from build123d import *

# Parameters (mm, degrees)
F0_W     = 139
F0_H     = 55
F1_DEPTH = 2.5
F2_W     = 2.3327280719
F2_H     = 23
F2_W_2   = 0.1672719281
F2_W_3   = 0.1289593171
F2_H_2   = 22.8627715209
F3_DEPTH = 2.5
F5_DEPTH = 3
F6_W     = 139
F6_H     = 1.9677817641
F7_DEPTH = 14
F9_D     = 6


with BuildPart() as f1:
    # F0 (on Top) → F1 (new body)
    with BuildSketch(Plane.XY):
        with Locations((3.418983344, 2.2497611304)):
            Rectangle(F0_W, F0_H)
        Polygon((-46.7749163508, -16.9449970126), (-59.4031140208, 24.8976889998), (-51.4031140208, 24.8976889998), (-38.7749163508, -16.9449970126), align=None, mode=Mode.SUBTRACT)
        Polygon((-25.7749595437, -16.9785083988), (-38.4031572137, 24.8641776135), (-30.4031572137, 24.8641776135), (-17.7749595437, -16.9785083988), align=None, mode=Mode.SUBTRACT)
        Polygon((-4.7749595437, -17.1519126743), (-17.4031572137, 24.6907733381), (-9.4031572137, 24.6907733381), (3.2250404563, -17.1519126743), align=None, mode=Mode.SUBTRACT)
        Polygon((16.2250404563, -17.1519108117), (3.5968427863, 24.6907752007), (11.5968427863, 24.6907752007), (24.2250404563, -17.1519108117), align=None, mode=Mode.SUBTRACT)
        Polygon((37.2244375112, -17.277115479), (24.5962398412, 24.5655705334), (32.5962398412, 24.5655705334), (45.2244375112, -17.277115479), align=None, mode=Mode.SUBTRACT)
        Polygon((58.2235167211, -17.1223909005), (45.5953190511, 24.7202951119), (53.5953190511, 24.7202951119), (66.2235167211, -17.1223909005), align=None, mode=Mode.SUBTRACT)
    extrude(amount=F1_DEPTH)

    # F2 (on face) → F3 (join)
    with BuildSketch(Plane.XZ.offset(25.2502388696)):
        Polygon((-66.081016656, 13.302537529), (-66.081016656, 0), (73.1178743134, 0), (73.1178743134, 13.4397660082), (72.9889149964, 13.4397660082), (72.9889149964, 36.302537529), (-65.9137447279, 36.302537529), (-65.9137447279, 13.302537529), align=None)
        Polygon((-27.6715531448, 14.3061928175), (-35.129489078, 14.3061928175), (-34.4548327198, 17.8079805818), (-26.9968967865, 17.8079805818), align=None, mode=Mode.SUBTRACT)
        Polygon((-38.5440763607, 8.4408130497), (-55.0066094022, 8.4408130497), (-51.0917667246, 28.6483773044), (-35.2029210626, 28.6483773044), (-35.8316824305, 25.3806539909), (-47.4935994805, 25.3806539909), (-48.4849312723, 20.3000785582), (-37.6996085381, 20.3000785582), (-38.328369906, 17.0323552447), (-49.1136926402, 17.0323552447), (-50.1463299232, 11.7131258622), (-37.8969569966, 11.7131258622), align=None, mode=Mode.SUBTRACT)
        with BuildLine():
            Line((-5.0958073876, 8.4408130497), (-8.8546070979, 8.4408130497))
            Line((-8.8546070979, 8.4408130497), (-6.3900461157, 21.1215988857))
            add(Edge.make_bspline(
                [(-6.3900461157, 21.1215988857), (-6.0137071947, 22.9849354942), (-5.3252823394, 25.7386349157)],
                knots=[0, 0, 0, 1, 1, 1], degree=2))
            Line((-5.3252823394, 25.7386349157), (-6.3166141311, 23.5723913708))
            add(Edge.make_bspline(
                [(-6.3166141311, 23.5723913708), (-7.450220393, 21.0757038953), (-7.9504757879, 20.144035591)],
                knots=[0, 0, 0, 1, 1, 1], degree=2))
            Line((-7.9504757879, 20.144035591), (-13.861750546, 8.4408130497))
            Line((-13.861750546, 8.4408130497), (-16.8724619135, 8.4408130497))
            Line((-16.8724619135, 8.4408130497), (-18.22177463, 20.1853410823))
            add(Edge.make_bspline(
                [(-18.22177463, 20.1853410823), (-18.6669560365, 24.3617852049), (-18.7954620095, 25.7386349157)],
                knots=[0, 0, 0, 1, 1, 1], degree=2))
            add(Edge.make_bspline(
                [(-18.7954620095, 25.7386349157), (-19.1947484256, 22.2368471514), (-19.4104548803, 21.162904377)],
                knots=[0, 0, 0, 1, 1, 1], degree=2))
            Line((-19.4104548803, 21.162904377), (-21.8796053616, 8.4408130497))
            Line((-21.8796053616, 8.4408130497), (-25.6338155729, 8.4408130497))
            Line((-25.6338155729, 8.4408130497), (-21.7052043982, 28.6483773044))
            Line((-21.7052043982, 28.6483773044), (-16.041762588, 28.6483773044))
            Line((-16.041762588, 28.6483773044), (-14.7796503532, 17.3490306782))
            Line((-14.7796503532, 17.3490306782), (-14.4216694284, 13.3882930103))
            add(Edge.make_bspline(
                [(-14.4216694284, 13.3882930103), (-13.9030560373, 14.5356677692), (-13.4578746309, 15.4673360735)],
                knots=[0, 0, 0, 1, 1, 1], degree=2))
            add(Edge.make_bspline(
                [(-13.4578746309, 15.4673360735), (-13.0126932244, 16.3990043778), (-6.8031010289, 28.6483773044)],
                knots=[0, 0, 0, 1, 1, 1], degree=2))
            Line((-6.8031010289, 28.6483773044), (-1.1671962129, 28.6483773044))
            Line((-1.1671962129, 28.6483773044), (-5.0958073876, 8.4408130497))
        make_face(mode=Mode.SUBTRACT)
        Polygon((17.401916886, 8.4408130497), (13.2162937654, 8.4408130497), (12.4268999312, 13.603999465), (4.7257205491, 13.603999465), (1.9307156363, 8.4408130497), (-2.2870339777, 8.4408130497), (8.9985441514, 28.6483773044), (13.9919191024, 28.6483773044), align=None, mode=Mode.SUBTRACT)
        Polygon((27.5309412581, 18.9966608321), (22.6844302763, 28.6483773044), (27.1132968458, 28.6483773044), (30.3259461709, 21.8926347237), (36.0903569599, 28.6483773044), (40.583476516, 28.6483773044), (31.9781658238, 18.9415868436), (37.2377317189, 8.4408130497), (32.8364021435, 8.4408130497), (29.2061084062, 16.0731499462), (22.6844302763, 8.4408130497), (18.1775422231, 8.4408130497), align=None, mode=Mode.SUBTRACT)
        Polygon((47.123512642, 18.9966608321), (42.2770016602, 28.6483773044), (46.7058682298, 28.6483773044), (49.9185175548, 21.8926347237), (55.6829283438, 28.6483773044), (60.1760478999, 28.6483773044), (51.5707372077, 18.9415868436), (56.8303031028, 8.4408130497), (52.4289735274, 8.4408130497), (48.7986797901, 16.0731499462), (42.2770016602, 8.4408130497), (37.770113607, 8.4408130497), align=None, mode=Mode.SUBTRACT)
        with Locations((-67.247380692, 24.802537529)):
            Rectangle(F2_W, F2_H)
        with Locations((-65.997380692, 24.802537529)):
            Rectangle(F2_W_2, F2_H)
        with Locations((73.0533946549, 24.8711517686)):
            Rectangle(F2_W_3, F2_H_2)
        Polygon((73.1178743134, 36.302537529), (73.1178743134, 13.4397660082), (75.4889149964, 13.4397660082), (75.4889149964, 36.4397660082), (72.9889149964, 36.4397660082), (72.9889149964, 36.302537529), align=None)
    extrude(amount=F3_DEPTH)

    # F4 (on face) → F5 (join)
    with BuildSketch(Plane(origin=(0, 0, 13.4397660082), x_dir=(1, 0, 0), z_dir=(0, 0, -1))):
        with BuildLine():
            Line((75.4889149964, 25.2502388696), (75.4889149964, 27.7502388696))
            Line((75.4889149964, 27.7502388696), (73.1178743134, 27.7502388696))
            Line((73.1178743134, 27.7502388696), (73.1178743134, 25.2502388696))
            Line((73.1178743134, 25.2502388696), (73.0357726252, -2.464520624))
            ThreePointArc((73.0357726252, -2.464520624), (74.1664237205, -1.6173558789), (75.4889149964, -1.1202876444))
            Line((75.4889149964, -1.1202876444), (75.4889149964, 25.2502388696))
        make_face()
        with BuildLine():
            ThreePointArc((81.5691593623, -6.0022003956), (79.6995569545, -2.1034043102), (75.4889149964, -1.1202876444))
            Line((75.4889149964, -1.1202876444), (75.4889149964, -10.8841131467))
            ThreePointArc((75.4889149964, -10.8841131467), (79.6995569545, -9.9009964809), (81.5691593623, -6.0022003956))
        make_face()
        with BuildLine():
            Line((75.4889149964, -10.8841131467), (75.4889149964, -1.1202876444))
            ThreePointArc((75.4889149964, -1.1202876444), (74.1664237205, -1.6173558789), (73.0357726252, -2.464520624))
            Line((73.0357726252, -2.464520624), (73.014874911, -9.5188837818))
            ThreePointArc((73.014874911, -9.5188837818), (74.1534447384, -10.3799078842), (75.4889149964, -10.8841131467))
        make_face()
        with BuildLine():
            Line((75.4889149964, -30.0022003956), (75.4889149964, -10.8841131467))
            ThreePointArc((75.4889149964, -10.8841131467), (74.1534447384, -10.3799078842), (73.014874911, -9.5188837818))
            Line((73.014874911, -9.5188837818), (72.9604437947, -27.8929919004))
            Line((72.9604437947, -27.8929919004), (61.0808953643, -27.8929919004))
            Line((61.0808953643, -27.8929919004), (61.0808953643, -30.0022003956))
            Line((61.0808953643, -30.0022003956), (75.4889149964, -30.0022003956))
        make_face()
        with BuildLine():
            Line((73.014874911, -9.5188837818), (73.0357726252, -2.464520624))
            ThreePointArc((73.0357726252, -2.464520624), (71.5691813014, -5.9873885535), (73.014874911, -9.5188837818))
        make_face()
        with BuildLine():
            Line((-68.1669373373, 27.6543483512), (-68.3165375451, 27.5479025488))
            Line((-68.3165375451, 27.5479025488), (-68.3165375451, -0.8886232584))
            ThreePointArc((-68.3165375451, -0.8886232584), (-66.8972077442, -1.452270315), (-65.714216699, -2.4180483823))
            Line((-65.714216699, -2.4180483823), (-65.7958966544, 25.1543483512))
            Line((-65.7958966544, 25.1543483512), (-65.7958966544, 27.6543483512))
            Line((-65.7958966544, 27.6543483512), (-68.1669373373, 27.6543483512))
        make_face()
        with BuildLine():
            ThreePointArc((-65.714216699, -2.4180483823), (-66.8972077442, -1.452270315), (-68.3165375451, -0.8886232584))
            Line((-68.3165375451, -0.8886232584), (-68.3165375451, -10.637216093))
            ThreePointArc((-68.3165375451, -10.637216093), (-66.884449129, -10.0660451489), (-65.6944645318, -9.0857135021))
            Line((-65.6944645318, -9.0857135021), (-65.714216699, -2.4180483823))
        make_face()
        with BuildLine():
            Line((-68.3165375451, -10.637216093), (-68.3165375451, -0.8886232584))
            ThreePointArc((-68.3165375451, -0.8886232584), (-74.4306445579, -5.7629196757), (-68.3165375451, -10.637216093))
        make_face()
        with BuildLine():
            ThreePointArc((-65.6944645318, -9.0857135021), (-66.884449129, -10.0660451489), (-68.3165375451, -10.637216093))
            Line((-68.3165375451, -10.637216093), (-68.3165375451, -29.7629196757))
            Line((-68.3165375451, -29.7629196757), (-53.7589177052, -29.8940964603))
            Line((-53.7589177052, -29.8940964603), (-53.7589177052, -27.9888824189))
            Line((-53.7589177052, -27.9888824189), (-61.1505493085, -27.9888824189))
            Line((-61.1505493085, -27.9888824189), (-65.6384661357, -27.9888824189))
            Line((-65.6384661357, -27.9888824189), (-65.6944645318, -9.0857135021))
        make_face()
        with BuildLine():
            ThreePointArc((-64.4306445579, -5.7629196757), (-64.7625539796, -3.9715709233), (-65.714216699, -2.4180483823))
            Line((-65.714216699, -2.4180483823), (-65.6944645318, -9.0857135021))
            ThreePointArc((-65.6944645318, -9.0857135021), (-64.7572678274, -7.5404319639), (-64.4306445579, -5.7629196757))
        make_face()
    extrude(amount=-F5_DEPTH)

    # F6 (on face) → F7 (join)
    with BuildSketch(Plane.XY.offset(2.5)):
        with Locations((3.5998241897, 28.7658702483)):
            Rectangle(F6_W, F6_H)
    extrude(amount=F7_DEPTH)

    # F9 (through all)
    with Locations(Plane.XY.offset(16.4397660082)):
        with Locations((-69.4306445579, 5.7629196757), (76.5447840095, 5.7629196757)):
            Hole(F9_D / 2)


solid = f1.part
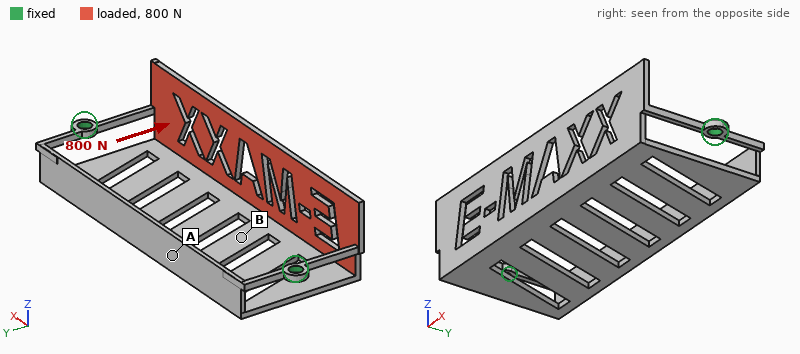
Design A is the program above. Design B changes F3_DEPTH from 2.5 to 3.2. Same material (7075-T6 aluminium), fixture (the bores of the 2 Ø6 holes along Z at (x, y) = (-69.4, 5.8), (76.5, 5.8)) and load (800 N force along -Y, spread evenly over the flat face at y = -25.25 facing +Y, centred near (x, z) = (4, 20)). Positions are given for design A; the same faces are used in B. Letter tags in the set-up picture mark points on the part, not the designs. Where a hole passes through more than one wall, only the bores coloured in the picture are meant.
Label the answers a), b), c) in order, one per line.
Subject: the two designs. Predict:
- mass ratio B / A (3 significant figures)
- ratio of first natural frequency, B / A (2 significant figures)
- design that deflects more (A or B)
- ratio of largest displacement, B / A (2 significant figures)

a) 1.10
b) 0.94
c) A
d) 0.73
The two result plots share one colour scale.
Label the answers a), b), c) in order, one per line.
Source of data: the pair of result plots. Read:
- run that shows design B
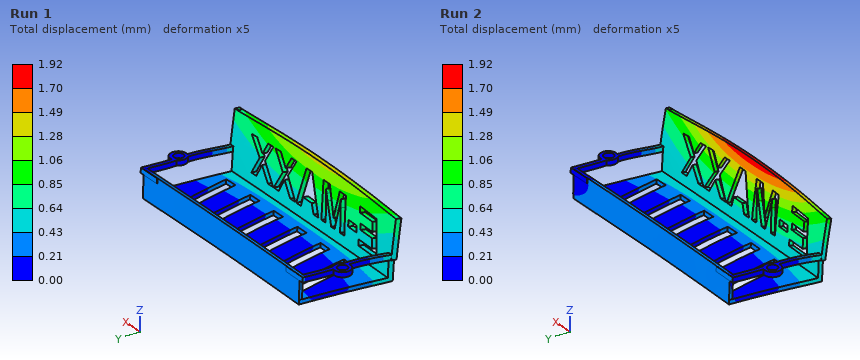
a) Run 1
